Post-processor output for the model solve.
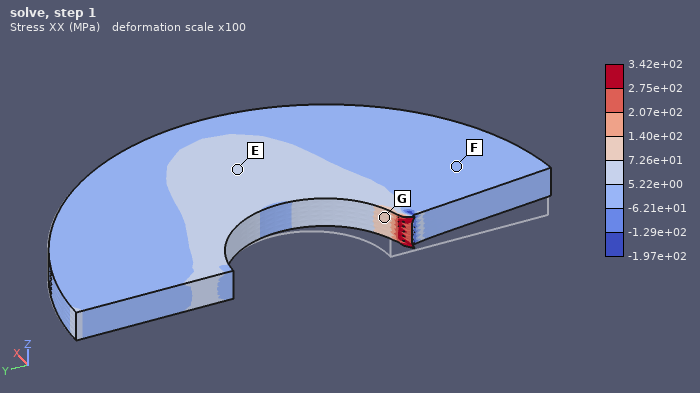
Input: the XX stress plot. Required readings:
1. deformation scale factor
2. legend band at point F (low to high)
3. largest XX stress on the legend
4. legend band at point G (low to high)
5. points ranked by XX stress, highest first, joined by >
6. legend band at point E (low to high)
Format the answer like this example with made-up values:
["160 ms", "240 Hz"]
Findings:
["100", "-6.21e+01 to 5.22e+00 MPa", "3.42e+02 MPa", "7.26e+01 to 1.40e+02 MPa", "G > E > F", "5.22e+00 to 7.26e+01 MPa"]
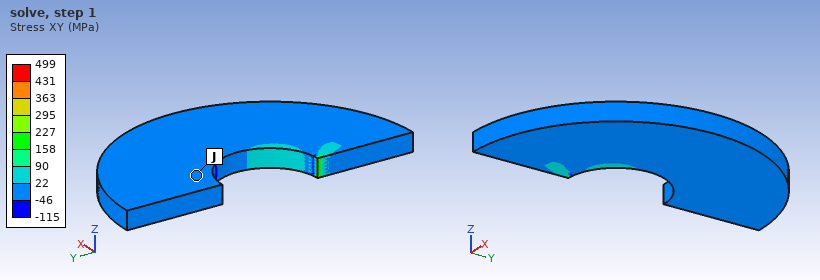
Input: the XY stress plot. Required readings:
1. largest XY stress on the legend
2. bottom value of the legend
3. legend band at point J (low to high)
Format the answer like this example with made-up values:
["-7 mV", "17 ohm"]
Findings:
["499 MPa", "-115 MPa", "-46 to 22 MPa"]
